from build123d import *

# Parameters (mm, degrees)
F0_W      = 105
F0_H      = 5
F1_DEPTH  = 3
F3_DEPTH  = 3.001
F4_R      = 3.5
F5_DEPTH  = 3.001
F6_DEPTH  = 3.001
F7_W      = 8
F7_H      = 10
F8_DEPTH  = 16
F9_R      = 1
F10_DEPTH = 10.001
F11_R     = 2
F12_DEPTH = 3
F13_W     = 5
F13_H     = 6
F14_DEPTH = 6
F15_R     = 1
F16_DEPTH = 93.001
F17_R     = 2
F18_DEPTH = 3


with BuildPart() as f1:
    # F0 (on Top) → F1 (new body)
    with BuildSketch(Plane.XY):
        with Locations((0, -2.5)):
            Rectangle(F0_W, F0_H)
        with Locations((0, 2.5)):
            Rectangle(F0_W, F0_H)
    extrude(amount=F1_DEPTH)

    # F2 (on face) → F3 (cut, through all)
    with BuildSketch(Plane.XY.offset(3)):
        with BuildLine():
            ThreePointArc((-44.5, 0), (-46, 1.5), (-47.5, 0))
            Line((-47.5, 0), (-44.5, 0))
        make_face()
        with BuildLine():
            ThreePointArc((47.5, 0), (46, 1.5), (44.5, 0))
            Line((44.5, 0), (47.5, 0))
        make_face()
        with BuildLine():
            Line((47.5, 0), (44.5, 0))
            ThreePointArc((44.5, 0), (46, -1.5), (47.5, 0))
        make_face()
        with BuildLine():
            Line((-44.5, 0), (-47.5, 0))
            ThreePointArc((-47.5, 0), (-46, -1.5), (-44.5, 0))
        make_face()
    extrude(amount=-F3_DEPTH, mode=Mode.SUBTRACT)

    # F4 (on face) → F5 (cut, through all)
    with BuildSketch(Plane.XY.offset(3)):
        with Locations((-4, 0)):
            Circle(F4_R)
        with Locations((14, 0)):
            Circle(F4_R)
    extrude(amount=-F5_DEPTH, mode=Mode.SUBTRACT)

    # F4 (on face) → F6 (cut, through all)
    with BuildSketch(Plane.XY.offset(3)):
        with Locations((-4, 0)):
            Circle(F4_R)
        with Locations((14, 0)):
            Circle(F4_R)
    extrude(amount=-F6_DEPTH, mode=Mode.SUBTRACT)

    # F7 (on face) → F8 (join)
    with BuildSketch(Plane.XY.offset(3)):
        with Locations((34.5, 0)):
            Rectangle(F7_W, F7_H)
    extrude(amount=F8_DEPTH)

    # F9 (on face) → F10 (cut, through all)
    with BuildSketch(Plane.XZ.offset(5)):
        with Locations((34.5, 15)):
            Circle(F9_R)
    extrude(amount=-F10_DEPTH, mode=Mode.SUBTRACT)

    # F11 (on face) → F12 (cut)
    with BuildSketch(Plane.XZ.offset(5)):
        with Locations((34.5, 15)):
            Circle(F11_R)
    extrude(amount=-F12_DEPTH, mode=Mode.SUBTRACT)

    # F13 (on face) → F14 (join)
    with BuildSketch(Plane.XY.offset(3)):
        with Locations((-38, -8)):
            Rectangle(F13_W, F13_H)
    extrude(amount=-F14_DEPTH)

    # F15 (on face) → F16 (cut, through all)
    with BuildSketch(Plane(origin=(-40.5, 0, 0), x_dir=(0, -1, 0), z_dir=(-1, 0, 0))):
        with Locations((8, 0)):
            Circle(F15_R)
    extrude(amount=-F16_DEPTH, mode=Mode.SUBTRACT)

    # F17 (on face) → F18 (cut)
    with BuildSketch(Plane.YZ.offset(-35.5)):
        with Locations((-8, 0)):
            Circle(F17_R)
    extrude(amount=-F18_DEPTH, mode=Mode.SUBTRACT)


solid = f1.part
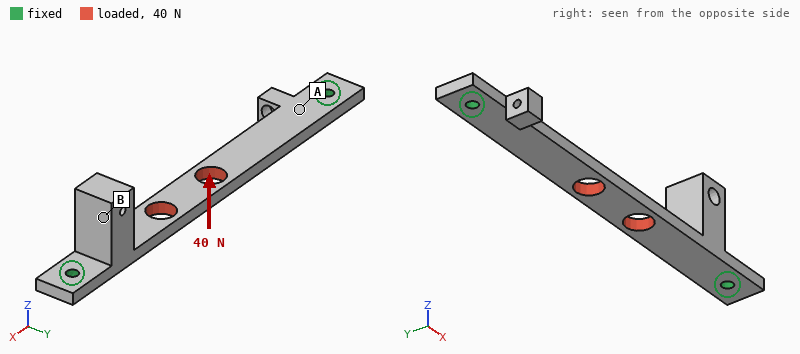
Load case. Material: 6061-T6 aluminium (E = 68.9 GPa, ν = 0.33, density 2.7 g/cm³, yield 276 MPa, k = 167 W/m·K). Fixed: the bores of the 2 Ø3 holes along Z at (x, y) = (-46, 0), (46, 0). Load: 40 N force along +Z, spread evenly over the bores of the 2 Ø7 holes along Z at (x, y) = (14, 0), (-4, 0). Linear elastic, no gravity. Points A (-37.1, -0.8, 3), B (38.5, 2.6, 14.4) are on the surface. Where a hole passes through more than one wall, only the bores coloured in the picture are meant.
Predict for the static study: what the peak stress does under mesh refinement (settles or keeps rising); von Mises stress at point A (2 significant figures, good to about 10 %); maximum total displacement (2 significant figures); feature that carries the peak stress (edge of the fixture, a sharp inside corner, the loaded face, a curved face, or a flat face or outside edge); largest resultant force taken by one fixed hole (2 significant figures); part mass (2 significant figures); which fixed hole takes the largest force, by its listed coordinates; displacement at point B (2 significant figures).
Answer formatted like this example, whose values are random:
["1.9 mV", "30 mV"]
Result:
["keeps rising", "17 MPa", "0.11 mm", "edge of the fixture", "25 N", "11 g", "(46, 0)", "0.035 mm"]
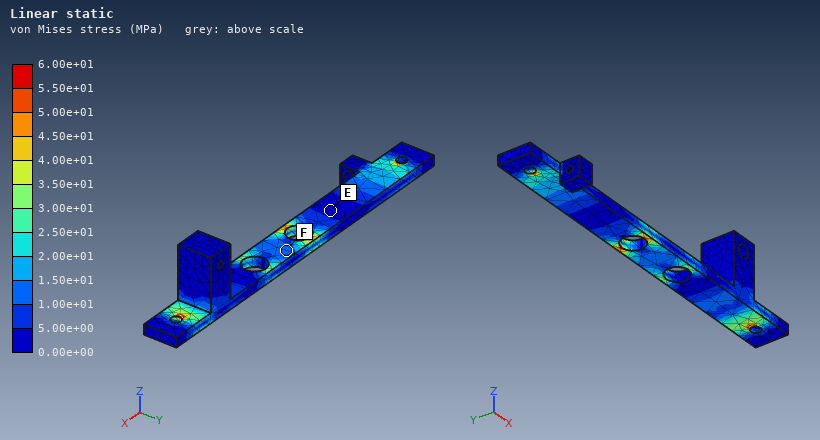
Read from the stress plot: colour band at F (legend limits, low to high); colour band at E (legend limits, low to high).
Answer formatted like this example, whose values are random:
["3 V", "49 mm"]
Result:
["1.00e+01 to 1.50e+01 MPa", "0.00e+00 to 5.00e+00 MPa"]
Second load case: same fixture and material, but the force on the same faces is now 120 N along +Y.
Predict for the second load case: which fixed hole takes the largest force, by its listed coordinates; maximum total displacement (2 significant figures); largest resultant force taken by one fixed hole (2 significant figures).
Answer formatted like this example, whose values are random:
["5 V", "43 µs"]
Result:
["(46, 0)", "43 µm", "69 N"]
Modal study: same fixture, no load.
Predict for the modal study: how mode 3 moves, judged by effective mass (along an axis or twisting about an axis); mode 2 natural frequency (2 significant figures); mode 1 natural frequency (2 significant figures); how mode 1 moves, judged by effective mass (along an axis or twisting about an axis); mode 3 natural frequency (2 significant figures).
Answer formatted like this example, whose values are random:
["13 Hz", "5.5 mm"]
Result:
["along Y", "3800 Hz", "1800 Hz", "along Z", "4100 Hz"]
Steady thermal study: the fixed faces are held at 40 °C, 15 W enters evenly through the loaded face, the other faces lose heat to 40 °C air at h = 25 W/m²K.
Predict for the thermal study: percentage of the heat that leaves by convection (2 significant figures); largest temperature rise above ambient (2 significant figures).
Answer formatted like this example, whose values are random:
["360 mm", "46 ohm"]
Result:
["12 %", "58 K"]
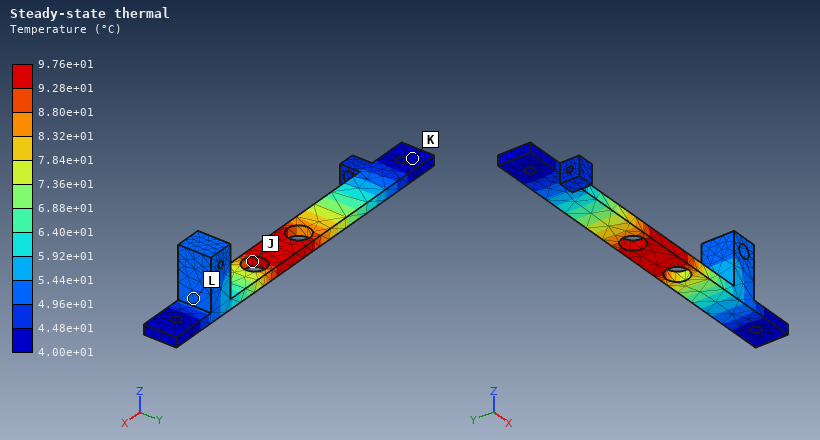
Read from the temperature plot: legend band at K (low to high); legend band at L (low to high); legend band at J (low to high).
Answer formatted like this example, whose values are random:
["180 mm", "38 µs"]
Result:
["4.00e+01 to 4.48e+01 °C", "4.96e+01 to 5.44e+01 °C", "9.28e+01 to 9.76e+01 °C"]
